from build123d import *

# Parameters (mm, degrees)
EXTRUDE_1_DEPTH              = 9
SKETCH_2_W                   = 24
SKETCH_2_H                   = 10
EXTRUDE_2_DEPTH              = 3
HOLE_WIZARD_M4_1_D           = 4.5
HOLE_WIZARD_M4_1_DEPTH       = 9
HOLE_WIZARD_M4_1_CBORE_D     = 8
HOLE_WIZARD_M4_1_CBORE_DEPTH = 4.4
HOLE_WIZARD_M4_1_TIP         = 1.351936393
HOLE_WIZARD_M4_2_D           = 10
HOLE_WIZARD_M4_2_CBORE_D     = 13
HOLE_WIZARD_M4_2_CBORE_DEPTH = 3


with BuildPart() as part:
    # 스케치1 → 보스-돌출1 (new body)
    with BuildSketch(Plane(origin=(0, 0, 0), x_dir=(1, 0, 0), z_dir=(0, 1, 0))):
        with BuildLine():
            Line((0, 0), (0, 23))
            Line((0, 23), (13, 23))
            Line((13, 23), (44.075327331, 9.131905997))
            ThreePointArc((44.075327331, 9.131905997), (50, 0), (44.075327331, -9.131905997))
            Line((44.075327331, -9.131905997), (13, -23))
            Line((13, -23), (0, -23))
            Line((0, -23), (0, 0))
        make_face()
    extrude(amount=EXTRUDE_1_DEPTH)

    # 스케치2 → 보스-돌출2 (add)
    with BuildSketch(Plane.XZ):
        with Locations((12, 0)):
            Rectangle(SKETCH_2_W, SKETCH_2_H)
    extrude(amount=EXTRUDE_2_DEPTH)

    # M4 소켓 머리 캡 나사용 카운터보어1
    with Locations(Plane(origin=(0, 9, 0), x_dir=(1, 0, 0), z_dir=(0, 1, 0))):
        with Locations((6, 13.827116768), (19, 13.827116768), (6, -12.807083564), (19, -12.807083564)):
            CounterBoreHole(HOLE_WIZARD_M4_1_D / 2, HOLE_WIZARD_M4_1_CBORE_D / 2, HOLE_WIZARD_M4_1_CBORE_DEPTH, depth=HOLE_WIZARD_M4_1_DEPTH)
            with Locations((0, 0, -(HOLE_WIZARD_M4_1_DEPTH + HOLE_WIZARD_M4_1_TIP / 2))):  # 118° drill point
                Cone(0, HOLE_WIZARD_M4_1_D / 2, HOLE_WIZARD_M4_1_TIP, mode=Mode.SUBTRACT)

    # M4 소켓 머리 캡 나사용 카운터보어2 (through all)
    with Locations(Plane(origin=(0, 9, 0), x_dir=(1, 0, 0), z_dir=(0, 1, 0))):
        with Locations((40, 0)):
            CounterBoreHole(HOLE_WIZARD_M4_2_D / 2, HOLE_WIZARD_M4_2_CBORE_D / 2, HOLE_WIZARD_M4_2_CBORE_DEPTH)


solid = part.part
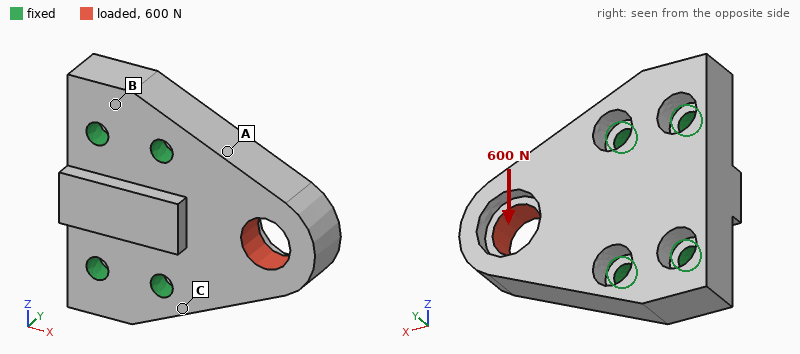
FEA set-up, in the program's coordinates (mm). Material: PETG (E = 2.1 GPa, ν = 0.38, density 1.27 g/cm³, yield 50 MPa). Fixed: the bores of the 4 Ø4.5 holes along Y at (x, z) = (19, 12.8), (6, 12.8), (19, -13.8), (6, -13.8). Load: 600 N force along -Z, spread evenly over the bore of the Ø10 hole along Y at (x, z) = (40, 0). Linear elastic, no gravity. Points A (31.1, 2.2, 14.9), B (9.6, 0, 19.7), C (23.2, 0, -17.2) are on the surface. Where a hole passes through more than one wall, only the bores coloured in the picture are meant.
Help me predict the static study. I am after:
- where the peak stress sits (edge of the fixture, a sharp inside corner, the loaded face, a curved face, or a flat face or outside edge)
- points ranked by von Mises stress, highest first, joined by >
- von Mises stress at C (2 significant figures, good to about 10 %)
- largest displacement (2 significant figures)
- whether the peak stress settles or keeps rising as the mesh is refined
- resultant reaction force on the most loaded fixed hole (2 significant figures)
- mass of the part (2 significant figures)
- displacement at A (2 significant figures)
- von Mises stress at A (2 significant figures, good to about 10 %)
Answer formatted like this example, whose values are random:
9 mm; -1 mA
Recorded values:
edge of the fixture; A > C > B; 4.8 MPa; 0.22 mm; keeps rising; 460 N; 17 g; 0.072 mm; 7.8 MPa
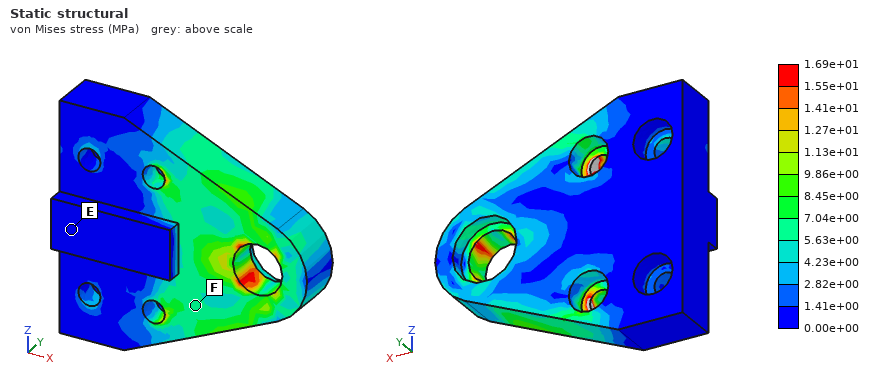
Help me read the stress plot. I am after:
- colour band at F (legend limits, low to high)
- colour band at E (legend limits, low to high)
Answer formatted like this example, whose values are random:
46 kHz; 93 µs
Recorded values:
5.63e+00 to 7.04e+00 MPa; 0.00e+00 to 1.41e+00 MPa
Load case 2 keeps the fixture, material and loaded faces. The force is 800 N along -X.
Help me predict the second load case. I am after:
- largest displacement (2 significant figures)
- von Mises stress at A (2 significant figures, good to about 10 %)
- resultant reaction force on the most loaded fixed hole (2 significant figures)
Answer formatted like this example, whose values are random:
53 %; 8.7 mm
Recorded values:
0.16 mm; 4.4 MPa; 320 N
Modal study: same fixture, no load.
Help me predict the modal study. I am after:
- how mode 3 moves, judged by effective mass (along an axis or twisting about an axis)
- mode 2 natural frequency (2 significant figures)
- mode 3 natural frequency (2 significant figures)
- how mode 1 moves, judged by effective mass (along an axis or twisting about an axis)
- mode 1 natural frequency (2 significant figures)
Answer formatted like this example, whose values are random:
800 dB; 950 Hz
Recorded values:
along Z; 5500 Hz; 5800 Hz; along Y; 2200 Hz
